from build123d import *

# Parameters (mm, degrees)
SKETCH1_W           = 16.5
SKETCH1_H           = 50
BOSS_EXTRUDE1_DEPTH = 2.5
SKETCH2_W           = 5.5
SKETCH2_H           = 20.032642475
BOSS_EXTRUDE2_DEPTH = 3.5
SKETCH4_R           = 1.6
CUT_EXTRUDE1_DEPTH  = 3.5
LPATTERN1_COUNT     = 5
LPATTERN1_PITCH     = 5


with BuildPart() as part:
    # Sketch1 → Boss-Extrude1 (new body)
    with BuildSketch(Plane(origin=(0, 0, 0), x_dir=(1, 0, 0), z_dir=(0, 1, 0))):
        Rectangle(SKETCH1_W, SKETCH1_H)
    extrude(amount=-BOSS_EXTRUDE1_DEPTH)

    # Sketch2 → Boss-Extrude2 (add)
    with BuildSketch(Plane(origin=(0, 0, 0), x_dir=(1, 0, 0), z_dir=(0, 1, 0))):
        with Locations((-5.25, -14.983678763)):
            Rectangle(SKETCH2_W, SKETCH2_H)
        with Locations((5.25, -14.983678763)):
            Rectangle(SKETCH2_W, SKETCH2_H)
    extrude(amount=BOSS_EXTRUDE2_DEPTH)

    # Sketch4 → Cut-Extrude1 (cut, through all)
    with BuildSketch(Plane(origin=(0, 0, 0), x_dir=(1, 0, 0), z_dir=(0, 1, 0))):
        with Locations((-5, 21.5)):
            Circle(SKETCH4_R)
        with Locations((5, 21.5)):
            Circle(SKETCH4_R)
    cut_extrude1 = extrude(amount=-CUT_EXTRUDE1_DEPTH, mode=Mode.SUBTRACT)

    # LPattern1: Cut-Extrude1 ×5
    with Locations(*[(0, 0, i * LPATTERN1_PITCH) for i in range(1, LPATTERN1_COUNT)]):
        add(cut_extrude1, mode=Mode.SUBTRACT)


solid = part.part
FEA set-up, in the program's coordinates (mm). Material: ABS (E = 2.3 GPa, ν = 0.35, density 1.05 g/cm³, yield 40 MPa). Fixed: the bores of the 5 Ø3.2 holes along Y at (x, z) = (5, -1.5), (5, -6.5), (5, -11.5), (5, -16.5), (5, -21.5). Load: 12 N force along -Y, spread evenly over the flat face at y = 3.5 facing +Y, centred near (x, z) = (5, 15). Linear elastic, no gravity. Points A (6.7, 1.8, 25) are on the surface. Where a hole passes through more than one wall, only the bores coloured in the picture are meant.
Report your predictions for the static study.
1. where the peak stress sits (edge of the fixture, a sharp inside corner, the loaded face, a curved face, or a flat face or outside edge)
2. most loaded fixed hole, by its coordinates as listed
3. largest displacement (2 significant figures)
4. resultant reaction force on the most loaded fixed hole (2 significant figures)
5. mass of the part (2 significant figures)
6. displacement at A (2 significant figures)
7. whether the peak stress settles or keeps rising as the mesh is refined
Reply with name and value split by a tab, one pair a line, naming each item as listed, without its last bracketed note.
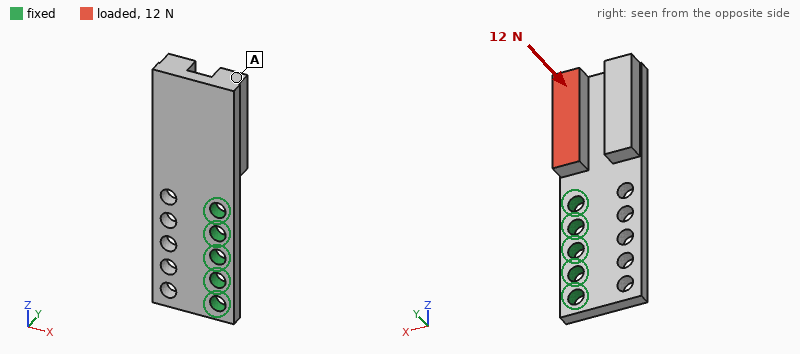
where the peak stress sits	edge of the fixture
most loaded fixed hole, by its coordinates as listed	(5, -1.5)
largest displacement	0.62 mm
resultant reaction force on the most loaded fixed hole	21 N
mass of the part	2.8 g
displacement at A	0.61 mm
whether the peak stress settles or keeps rising as the mesh is refined	keeps rising
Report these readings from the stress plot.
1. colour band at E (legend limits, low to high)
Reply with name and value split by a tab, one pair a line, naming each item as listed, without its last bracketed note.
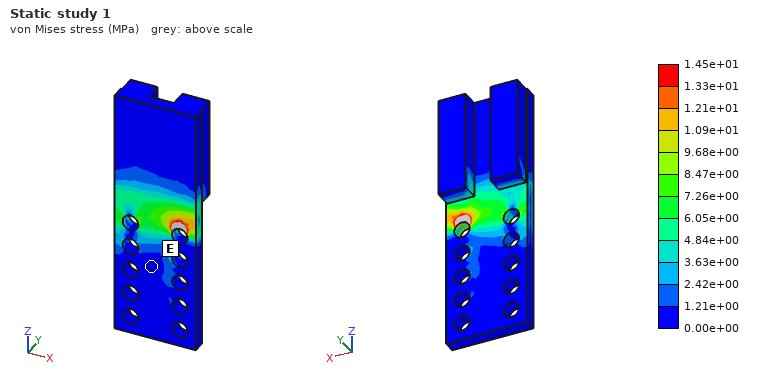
colour band at E	0.00e+00 to 1.21e+00 MPa
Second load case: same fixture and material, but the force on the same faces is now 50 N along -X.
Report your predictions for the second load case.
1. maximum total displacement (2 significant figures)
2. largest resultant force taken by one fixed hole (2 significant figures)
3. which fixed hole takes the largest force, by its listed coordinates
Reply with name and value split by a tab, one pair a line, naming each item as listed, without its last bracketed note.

maximum total displacement	0.51 mm
largest resultant force taken by one fixed hole	100 N
which fixed hole takes the largest force, by its listed coordinates	(5, -1.5)
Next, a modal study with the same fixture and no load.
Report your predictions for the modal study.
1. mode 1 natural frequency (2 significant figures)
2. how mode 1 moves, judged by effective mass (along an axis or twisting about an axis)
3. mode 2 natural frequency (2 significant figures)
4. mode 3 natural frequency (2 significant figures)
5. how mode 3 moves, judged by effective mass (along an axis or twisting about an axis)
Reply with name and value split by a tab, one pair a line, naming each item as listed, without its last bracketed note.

mode 1 natural frequency	630 Hz
how mode 1 moves, judged by effective mass	along Y
mode 2 natural frequency	1900 Hz
mode 3 natural frequency	2400 Hz
how mode 3 moves, judged by effective mass	along X
